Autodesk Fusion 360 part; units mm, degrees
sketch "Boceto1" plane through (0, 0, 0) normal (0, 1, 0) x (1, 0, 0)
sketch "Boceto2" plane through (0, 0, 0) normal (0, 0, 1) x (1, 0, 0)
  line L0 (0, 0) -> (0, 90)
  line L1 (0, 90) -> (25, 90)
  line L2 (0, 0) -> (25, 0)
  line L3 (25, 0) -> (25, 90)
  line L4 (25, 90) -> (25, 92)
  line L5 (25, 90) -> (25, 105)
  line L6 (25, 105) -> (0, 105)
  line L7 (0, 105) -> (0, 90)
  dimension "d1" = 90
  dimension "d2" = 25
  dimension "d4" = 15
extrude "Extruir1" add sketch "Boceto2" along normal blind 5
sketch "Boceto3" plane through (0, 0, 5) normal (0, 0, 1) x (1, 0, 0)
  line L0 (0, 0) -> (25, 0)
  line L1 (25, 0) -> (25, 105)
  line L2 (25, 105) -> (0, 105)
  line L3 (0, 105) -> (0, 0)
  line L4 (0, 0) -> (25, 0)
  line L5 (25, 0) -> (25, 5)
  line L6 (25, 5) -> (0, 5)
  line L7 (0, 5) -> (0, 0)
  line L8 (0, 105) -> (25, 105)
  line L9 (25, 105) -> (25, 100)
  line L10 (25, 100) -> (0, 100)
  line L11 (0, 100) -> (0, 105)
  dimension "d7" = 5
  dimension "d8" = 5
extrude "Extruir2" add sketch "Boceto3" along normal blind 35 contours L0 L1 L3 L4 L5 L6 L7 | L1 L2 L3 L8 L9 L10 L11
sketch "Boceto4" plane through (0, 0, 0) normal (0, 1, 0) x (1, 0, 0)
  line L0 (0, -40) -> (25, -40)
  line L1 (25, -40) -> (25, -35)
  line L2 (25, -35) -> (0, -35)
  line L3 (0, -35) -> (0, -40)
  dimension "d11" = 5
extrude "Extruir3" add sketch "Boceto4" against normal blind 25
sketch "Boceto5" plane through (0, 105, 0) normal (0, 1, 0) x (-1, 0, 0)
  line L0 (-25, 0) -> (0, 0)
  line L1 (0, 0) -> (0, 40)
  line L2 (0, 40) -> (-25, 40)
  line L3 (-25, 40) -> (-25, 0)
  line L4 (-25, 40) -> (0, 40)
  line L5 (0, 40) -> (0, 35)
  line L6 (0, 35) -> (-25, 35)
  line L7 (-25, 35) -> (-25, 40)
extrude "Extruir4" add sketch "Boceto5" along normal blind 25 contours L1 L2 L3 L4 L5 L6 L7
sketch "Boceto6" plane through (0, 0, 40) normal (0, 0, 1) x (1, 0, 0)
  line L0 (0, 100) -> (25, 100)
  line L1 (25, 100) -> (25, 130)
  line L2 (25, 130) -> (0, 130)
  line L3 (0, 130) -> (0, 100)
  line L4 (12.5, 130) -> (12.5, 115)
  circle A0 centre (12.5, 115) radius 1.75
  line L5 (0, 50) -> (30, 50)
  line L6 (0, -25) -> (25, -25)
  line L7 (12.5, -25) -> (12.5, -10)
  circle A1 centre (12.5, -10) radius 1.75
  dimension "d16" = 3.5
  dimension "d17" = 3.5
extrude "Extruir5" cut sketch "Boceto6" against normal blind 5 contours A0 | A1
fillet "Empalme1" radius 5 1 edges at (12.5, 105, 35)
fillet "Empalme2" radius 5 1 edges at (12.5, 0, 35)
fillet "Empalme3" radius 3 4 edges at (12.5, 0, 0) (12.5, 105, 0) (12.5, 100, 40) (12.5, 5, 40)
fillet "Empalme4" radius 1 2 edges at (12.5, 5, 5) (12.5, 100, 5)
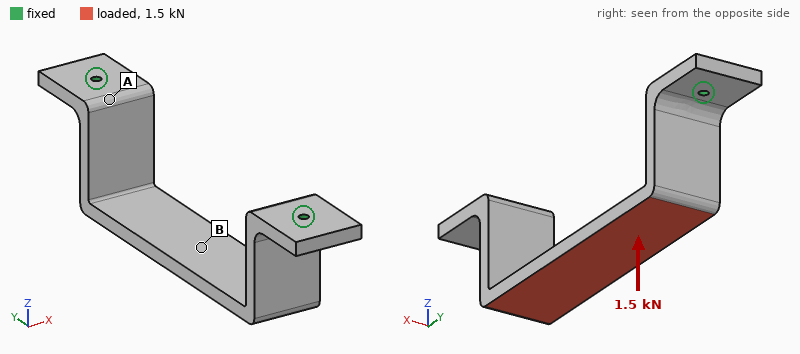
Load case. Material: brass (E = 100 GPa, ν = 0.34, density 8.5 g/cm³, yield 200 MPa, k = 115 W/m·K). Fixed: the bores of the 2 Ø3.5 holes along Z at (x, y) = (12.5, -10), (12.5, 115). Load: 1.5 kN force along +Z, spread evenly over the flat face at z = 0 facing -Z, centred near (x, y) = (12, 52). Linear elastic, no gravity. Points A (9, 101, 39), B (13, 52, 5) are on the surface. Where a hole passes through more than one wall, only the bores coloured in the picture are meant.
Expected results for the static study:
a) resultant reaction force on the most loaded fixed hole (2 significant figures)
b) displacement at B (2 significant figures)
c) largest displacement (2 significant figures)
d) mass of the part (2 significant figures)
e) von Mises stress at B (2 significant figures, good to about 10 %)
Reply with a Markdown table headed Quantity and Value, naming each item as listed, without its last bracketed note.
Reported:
| Quantity | Value |
|---|---|
| resultant reaction force on the most loaded fixed hole | 910 N |
| displacement at B | 0.22 mm |
| largest displacement | 0.22 mm |
| mass of the part | 240 g |
| von Mises stress at B | 66 MPa |
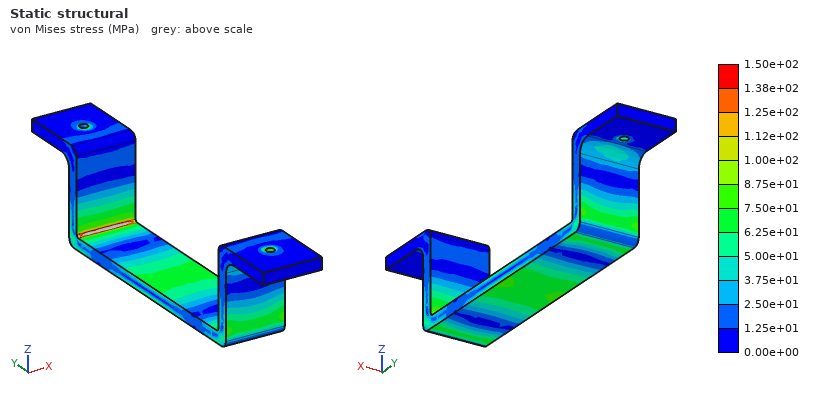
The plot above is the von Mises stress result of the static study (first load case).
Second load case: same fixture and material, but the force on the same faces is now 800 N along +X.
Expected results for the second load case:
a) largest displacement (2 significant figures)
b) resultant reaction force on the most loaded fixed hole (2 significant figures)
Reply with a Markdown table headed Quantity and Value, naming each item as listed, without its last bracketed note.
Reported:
| Quantity | Value |
|---|---|
| largest displacement | 0.20 mm |
| resultant reaction force on the most loaded fixed hole | 400 N |
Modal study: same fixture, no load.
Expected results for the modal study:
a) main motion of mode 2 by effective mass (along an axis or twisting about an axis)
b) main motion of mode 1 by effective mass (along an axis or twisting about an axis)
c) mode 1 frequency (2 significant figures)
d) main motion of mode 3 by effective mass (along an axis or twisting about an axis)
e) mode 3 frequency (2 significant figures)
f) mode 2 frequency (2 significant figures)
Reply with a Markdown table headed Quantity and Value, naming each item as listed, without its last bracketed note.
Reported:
| Quantity | Value |
|---|---|
| main motion of mode 2 by effective mass | along Y |
| main motion of mode 1 by effective mass | along X |
| mode 1 frequency | 960 Hz |
| main motion of mode 3 by effective mass | along Z |
| mode 3 frequency | 1500 Hz |
| mode 2 frequency | 1000 Hz |
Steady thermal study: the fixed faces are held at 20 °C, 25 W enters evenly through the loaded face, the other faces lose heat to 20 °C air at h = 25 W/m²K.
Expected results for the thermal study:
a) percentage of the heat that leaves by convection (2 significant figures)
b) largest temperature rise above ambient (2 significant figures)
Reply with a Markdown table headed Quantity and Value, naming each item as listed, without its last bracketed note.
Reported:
| Quantity | Value |
|---|---|
| percentage of the heat that leaves by convection | 24 % |
| largest temperature rise above ambient | 49 K |
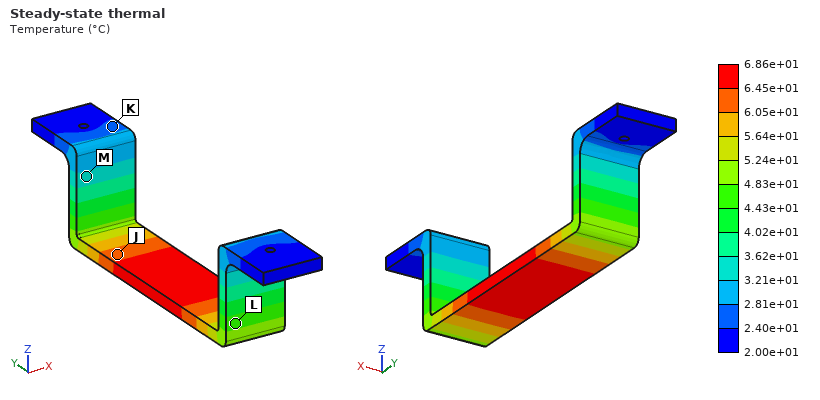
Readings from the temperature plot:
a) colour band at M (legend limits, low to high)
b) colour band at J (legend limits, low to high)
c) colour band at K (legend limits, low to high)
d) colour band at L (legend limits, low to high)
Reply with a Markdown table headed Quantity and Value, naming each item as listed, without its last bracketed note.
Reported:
| Quantity | Value |
|---|---|
| colour band at M | 3.21e+01 to 3.62e+01 °C |
| colour band at J | 6.05e+01 to 6.45e+01 °C |
| colour band at K | 2.40e+01 to 2.81e+01 °C |
| colour band at L | 4.43e+01 to 4.83e+01 °C |
